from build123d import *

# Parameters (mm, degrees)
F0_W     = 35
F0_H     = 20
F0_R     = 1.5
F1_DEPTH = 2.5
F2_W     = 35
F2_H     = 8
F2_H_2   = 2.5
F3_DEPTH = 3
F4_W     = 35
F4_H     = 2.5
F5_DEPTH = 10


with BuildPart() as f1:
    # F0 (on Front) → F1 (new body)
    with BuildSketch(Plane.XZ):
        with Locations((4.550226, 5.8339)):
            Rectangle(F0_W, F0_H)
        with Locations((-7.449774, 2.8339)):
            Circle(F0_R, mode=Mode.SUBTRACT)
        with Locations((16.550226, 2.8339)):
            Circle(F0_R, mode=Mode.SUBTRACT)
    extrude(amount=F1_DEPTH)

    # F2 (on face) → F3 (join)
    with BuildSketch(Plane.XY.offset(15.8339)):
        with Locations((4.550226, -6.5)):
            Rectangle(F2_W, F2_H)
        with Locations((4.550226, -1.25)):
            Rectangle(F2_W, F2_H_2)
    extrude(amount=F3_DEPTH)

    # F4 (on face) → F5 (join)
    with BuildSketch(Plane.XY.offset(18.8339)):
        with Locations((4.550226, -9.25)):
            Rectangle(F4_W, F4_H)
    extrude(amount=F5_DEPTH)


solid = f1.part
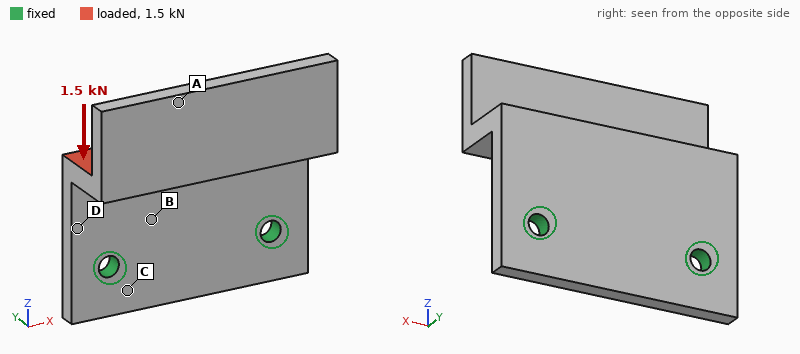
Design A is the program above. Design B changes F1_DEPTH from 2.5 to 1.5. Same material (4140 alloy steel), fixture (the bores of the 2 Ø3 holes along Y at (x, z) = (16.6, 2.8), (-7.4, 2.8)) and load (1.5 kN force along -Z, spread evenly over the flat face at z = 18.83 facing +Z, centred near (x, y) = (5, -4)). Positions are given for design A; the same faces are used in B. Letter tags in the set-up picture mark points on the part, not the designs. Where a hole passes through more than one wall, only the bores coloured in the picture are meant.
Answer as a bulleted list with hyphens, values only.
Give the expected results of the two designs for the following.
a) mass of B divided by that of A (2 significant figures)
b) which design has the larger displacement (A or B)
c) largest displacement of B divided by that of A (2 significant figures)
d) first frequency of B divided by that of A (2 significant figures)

- 0.81
- B
- 5.1
- 0.48
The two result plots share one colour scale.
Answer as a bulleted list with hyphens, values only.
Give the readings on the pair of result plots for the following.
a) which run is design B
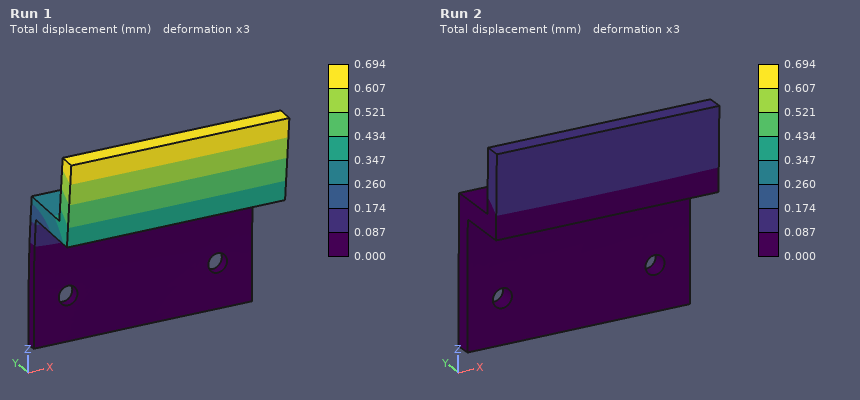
- Run 1
